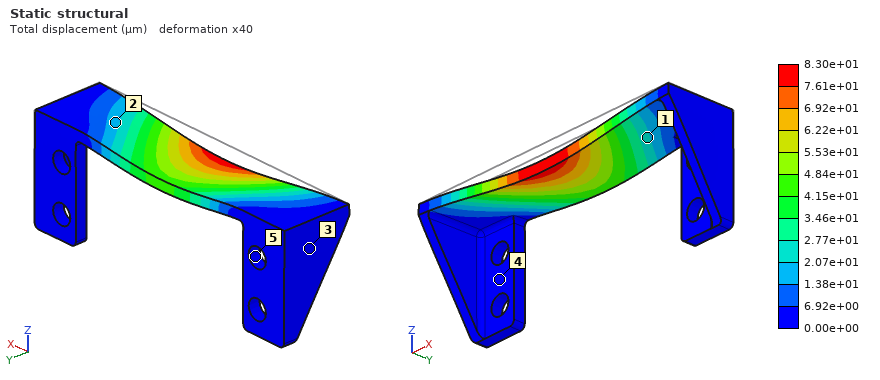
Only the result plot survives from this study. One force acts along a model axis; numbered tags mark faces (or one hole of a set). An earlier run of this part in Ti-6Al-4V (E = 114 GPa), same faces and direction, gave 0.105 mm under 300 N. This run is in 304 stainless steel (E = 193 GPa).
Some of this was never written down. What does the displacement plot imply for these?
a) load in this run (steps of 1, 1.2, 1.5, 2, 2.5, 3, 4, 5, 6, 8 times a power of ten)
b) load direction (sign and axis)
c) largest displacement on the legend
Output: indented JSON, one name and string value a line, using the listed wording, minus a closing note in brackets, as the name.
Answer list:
{
  "load in this run": "400 N",
  "load direction": "-Z",
  "largest displacement on the legend": "8.30e+01 µm"
}
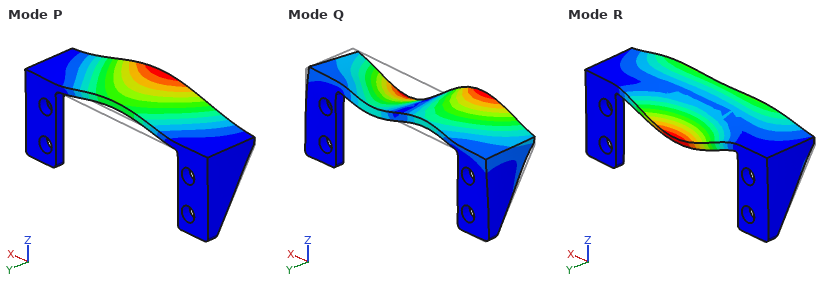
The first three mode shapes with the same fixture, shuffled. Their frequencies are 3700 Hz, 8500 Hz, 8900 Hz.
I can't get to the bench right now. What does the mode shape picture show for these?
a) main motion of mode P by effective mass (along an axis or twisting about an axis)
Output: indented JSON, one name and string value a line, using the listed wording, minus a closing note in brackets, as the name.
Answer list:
{
  "main motion of mode P by effective mass": "along Z"
}
